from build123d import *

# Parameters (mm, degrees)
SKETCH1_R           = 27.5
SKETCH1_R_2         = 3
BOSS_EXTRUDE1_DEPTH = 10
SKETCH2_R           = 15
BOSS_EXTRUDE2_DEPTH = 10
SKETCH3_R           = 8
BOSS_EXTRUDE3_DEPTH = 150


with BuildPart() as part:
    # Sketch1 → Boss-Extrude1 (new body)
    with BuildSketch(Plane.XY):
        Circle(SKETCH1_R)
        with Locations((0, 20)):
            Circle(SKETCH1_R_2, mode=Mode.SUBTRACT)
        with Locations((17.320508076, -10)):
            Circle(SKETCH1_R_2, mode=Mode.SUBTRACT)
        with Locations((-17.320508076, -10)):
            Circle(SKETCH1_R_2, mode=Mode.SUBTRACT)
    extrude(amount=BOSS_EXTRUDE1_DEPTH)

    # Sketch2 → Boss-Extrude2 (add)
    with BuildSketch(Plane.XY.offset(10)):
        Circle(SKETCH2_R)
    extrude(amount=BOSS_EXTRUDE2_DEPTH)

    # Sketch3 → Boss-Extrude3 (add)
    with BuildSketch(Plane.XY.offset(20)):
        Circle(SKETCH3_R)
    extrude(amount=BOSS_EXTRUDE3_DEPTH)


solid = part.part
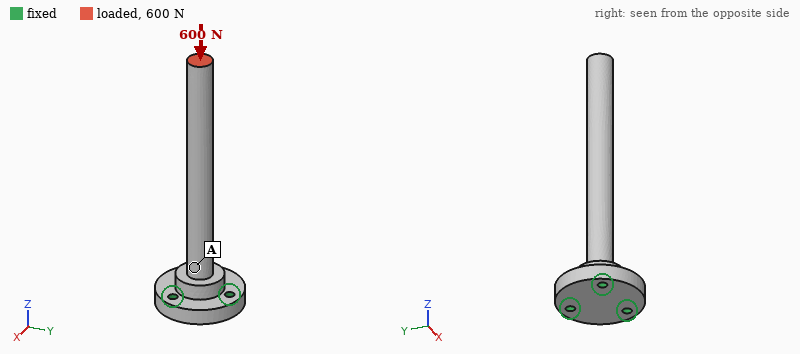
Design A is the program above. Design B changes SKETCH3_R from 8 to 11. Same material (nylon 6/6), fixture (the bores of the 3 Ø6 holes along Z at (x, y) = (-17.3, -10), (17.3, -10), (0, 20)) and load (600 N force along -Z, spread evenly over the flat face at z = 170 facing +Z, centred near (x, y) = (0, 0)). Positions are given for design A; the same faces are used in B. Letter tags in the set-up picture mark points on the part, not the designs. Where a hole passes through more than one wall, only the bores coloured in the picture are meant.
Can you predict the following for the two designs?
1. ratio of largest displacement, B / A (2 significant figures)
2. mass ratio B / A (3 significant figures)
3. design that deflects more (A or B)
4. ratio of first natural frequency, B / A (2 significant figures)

0.56
1.45
A
1.3
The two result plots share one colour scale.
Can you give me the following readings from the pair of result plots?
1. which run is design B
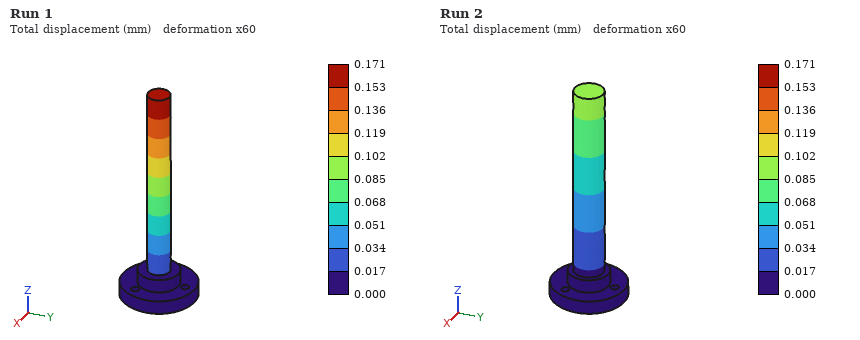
Run 2
